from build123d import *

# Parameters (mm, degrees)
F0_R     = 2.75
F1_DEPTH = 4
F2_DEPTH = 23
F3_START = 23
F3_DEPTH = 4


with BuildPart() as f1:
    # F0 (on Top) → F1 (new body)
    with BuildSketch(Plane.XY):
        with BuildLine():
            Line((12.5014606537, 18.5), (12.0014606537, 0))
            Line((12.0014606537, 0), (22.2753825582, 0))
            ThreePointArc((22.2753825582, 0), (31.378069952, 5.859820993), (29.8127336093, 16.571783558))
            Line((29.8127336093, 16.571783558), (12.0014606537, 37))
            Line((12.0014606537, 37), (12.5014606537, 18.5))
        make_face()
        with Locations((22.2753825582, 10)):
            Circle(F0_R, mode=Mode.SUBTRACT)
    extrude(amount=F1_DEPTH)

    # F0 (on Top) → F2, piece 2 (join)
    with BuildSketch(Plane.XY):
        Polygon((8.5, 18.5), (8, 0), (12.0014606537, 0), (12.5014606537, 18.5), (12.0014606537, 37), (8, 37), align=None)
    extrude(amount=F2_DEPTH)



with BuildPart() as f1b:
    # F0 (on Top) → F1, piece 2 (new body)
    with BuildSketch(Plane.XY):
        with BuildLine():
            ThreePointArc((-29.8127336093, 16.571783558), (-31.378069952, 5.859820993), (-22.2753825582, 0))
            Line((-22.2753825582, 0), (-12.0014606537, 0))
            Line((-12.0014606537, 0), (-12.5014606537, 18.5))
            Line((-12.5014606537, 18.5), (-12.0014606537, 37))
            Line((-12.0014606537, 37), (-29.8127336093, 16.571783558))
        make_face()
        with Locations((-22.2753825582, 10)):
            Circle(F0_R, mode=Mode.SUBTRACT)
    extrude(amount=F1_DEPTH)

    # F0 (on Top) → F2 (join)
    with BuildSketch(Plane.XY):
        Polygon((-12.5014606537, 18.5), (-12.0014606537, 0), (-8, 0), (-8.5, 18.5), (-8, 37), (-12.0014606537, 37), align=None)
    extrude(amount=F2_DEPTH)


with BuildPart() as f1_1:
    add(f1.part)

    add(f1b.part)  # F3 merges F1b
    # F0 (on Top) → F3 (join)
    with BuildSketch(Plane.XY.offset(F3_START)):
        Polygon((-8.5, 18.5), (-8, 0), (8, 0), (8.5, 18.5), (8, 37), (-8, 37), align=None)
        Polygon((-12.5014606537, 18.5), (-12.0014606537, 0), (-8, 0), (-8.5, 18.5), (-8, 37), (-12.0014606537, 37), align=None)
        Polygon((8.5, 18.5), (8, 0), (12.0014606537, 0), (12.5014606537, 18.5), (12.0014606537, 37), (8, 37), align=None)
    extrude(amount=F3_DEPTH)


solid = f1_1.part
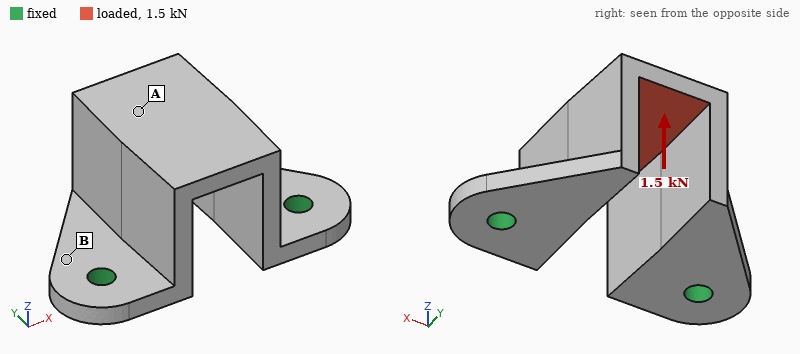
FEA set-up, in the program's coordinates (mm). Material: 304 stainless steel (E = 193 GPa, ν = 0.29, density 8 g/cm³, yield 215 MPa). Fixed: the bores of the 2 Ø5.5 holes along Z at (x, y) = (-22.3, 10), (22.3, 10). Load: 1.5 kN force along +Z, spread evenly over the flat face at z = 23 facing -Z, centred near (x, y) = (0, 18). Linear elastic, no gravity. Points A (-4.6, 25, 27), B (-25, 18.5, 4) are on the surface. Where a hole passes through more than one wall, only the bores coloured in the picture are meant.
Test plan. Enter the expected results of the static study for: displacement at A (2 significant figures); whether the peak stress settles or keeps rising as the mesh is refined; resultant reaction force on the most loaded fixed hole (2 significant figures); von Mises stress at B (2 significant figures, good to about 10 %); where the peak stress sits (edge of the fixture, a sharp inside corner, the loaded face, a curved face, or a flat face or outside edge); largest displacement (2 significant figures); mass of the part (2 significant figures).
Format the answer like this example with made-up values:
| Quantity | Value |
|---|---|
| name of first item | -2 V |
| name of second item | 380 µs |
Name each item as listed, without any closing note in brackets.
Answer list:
| Quantity | Value |
|---|---|
| displacement at A | 42 µm |
| whether the peak stress settles or keeps rising as the mesh is refined | keeps rising |
| resultant reaction force on the most loaded fixed hole | 810 N |
| von Mises stress at B | 54 MPa |
| where the peak stress sits | edge of the fixture |
| largest displacement | 54 µm |
| mass of the part | 110 g |
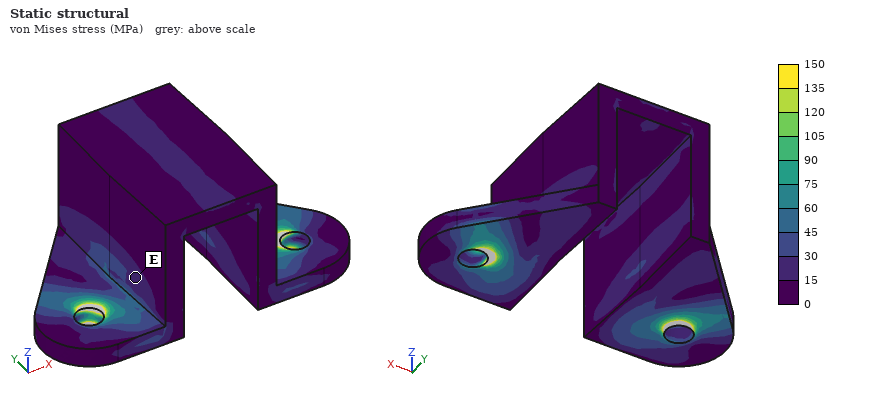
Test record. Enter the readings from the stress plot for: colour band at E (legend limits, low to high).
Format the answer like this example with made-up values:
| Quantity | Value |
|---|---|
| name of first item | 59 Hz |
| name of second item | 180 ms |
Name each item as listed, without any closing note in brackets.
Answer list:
| Quantity | Value |
|---|---|
| colour band at E | 15 to 30 MPa |
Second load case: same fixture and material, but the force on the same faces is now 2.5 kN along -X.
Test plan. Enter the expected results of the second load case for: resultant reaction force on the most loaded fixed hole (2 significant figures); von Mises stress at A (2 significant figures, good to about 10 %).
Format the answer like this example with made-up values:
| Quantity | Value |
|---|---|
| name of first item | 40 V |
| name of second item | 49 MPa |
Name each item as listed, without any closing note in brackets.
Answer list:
| Quantity | Value |
|---|---|
| resultant reaction force on the most loaded fixed hole | 1.8 kN |
| von Mises stress at A | 60 MPa |
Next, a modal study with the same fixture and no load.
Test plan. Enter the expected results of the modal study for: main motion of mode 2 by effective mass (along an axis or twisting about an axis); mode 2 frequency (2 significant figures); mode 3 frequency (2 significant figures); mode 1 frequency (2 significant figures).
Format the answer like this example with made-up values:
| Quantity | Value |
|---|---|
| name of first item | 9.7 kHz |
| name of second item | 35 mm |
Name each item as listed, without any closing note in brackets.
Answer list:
| Quantity | Value |
|---|---|
| main motion of mode 2 by effective mass | along X |
| mode 2 frequency | 4700 Hz |
| mode 3 frequency | 6300 Hz |
| mode 1 frequency | 2400 Hz |
